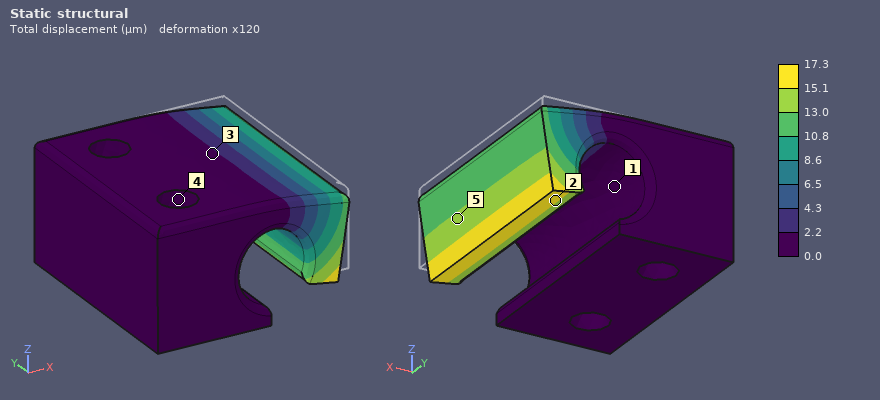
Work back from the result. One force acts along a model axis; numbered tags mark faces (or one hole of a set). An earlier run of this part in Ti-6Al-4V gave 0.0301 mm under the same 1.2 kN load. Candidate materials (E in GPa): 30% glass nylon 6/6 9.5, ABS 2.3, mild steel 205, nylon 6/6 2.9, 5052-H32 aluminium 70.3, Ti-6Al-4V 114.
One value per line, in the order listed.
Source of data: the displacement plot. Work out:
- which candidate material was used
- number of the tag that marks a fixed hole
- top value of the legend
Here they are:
mild steel
4
17.3 µm
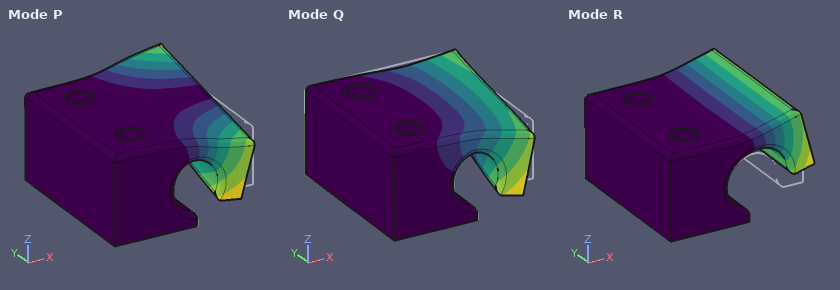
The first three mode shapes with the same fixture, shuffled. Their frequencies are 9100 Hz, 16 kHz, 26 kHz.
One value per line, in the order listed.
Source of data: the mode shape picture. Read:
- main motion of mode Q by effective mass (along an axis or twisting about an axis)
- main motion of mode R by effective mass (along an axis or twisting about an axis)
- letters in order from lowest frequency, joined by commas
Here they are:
along Y
along Z
R, P, Q
